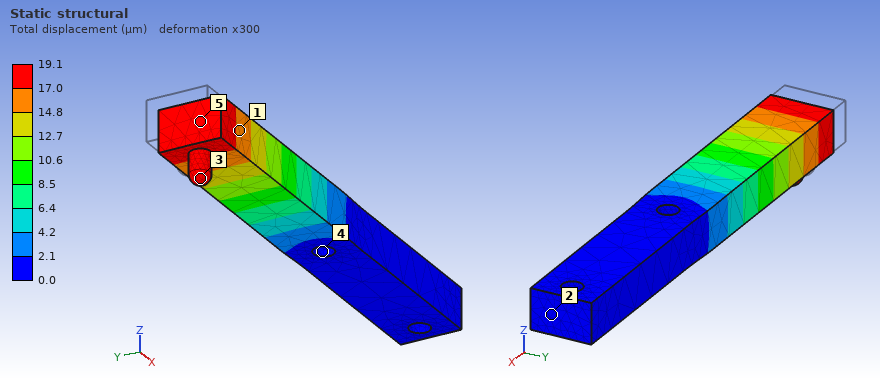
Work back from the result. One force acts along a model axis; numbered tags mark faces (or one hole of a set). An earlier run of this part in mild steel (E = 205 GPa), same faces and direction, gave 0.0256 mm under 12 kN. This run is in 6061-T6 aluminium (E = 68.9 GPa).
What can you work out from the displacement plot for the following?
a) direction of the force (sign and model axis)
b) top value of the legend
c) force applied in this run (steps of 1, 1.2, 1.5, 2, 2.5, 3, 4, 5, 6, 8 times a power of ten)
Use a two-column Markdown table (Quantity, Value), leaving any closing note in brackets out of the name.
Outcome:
| Quantity | Value |
|---|---|
| direction of the force | +X |
| top value of the legend | 19.1 µm |
| force applied in this run | 3 kN |
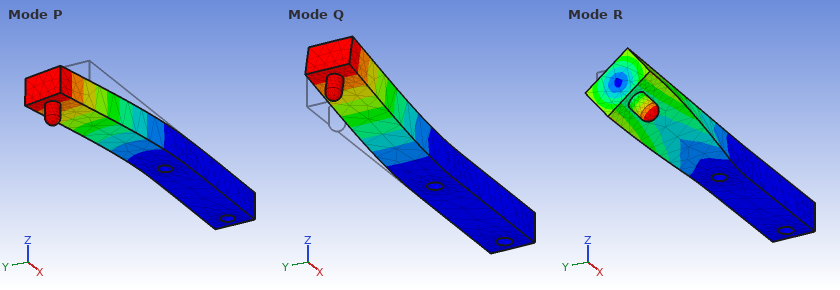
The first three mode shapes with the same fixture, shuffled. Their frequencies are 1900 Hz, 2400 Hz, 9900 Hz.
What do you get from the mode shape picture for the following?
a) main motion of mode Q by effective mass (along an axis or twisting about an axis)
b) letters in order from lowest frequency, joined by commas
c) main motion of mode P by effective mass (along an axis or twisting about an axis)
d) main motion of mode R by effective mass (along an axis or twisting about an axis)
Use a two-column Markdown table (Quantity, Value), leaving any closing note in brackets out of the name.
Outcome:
| Quantity | Value |
|---|---|
| main motion of mode Q by effective mass | along Z |
| letters in order from lowest frequency, joined by commas | Q, P, R |
| main motion of mode P by effective mass | along Y |
| main motion of mode R by effective mass | twisting about X |
